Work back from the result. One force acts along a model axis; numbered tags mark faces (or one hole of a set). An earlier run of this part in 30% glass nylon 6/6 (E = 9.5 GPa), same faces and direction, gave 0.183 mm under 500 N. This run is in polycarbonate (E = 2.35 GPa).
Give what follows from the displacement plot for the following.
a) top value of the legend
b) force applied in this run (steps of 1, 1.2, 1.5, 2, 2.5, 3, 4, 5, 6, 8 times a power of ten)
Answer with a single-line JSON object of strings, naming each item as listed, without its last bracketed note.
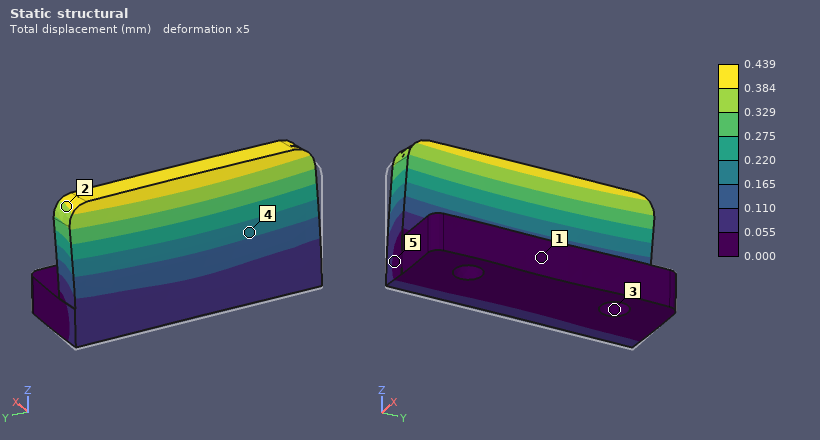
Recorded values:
{"top value of the legend": "0.439 mm", "force applied in this run": "300 N"}
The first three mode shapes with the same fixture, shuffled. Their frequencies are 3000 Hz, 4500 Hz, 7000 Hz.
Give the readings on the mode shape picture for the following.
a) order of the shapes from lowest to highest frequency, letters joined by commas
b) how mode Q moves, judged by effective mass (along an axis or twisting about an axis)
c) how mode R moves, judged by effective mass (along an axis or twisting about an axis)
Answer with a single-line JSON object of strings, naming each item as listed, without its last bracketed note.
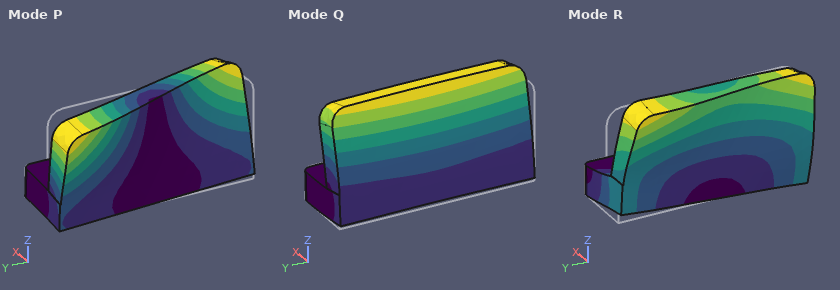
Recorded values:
{"order of the shapes from lowest to highest frequency, letters joined by commas": "Q, P, R", "how mode Q moves, judged by effective mass": "along X", "how mode R moves, judged by effective mass": "along Y"}
